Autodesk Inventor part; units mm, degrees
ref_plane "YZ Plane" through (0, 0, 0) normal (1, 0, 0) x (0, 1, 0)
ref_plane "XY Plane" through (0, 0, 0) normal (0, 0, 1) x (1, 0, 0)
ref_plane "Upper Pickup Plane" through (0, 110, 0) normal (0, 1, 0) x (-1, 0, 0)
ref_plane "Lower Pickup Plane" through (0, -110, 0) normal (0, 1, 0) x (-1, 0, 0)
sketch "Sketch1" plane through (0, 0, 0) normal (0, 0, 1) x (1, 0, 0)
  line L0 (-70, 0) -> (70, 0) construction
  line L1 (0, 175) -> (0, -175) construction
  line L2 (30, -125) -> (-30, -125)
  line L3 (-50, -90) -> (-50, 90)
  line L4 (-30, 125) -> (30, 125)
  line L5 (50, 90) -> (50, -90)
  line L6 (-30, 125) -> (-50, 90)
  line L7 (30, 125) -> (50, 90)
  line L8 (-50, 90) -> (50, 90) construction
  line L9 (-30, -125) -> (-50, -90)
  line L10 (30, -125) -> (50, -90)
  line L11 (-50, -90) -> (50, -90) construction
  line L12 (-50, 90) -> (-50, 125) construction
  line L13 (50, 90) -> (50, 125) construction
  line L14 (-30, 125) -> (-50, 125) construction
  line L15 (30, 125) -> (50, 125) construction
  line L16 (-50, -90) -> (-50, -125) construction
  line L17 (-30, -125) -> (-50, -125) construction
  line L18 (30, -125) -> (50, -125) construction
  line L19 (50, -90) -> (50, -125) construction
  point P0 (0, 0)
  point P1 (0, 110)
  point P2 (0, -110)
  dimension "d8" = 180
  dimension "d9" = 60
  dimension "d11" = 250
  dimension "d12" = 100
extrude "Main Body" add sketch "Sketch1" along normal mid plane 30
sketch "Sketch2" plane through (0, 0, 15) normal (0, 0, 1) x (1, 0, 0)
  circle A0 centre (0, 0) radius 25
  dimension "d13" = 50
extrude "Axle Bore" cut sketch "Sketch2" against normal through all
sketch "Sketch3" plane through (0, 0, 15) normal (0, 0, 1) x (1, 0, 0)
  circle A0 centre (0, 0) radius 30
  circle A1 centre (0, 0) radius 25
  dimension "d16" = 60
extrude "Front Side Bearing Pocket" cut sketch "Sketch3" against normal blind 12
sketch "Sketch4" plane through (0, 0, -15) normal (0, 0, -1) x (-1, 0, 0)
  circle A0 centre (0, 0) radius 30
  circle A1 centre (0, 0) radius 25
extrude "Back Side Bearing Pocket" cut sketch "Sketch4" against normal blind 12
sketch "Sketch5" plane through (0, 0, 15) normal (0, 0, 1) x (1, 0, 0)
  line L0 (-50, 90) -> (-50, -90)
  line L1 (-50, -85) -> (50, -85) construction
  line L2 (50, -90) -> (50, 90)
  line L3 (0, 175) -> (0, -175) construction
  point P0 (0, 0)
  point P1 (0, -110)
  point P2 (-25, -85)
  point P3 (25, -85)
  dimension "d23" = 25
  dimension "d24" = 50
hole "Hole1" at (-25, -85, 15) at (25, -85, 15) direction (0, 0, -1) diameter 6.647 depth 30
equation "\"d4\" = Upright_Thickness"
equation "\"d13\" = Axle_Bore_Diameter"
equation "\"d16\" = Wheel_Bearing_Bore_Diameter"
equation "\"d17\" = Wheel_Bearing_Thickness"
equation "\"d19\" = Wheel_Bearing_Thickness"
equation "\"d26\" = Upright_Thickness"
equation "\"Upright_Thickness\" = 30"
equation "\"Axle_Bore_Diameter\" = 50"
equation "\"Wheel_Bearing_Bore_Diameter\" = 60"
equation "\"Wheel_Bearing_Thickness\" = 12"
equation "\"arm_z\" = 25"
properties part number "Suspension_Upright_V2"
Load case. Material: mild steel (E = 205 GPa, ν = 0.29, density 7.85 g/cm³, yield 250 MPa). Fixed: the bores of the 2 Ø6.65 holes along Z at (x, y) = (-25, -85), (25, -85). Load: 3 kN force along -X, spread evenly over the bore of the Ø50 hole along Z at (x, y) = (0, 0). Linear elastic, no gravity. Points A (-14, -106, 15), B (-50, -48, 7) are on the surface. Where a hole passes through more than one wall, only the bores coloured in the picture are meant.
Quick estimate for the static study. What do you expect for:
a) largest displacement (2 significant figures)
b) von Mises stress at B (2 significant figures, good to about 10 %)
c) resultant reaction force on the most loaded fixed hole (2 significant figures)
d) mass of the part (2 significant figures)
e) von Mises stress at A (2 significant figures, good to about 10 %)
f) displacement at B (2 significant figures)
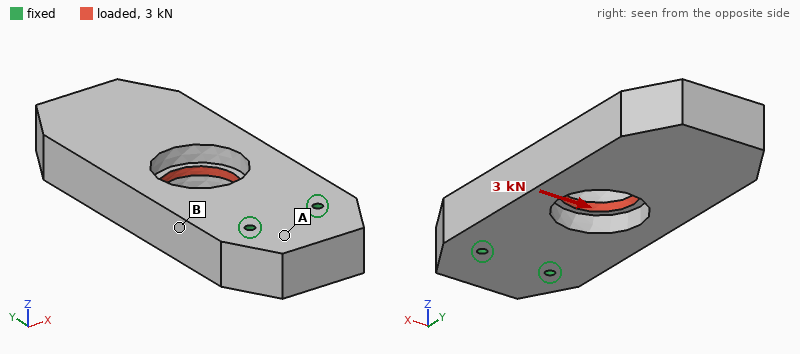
11 µm
3.9 MPa
5.0 kN
4.9 kg
1.2 MPa
2.3 µm
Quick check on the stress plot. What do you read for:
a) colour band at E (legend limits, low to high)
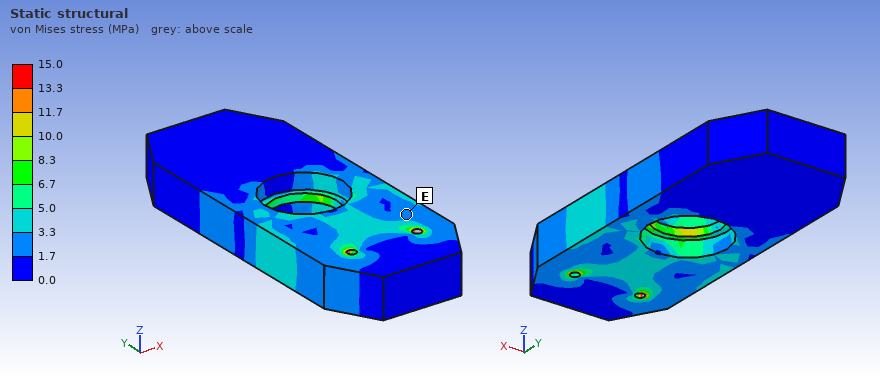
1.7 to 3.3 MPa
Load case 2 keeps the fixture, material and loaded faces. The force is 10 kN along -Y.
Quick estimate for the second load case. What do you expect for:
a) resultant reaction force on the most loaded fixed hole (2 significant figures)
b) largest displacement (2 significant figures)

5.0 kN
3.4 µm
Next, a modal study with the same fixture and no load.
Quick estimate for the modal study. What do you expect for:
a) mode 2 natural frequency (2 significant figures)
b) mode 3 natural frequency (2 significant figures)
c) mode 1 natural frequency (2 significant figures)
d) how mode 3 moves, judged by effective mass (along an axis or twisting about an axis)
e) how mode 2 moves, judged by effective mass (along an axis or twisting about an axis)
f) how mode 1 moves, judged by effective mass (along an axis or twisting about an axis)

1300 Hz
1900 Hz
480 Hz
twisting about Y
along X
along Z
